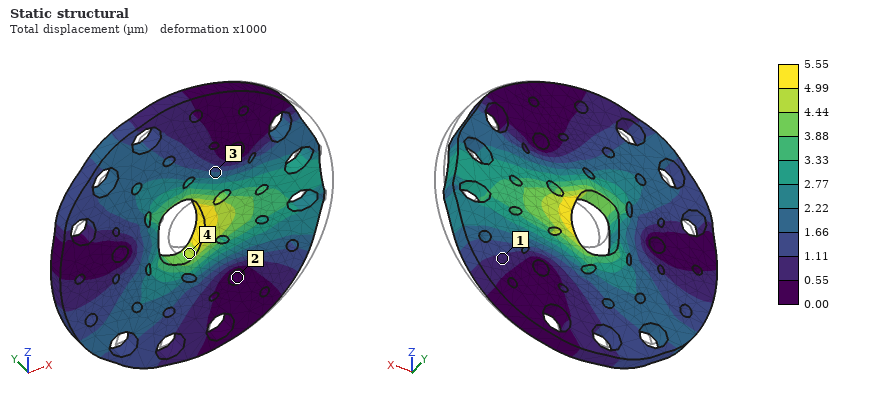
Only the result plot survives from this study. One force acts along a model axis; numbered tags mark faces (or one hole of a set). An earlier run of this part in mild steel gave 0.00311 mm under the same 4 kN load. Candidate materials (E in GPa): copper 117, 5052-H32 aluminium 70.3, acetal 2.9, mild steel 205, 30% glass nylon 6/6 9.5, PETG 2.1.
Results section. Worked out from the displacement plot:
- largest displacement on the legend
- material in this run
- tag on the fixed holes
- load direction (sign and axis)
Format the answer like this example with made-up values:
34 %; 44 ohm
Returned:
5.55 µm; copper; 2; -X
